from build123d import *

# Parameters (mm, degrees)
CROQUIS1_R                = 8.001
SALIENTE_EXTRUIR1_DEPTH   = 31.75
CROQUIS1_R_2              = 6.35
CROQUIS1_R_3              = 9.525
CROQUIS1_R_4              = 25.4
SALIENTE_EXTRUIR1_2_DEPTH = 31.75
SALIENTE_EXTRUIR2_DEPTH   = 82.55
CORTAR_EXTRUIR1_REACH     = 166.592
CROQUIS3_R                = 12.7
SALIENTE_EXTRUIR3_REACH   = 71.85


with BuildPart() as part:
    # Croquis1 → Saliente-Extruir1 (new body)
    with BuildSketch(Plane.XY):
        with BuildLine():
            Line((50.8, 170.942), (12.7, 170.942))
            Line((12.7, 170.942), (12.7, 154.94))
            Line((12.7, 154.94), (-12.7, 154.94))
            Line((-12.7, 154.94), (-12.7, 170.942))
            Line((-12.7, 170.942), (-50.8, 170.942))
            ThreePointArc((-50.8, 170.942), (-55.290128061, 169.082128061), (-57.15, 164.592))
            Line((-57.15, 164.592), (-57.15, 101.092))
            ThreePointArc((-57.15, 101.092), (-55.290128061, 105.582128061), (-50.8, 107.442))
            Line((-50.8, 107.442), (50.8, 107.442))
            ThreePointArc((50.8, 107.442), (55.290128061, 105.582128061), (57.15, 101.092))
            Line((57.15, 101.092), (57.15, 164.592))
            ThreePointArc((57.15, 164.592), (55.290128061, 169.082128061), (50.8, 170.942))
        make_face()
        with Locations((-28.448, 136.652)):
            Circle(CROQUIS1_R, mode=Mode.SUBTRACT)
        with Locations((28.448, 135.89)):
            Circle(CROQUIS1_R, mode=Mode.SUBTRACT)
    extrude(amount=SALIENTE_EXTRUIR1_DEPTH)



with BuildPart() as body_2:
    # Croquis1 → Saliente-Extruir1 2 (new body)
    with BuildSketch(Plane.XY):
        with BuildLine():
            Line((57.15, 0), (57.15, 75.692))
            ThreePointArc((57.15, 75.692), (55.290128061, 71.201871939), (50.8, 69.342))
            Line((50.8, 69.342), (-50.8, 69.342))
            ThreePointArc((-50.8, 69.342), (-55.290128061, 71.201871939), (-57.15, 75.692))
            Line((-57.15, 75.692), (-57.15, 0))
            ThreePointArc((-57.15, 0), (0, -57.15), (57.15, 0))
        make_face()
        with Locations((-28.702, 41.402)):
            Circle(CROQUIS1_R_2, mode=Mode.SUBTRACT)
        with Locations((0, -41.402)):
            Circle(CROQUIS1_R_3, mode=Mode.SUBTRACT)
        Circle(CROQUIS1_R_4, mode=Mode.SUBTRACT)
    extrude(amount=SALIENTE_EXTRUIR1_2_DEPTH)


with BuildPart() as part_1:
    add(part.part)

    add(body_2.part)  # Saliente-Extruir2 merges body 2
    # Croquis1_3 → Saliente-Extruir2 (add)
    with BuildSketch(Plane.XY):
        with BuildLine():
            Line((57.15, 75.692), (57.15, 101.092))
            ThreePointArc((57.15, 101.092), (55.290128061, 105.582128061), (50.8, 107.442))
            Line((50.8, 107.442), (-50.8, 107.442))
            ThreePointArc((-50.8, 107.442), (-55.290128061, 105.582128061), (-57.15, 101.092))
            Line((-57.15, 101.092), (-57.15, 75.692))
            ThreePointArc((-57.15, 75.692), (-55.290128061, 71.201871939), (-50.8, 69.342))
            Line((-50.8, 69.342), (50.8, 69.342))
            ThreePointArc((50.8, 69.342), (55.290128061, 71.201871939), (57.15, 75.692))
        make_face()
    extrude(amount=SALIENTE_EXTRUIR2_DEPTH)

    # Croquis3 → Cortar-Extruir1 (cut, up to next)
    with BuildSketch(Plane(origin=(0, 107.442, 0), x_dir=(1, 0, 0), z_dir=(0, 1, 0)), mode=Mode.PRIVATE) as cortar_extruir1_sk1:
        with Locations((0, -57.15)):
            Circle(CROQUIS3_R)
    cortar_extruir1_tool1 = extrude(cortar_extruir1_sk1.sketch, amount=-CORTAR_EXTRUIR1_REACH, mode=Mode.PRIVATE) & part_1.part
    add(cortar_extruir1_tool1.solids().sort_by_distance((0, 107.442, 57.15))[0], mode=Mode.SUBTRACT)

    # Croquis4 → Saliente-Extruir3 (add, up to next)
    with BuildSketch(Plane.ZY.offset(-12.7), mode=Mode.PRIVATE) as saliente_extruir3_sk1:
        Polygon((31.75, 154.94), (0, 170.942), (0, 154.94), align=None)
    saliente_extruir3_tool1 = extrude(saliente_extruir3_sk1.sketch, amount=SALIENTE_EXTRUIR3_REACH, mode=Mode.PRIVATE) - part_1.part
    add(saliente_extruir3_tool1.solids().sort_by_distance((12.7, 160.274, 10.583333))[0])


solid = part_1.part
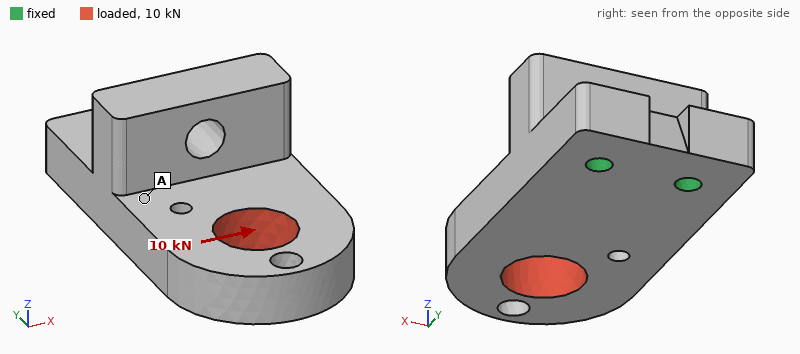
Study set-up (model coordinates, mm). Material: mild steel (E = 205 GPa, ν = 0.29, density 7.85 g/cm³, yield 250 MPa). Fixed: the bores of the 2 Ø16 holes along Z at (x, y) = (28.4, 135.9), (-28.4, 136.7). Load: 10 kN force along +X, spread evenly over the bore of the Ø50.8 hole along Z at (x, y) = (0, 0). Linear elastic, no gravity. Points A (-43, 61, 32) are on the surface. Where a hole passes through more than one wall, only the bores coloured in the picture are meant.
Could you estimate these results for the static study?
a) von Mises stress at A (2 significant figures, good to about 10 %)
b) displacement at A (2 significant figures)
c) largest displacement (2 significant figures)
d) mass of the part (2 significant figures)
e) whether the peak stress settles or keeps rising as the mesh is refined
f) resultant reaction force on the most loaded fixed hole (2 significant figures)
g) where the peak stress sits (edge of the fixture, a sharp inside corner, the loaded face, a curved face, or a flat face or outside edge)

7.1 MPa
9.3 µm
31 µm
7.0 kg
keeps rising
21 kN
edge of the fixture
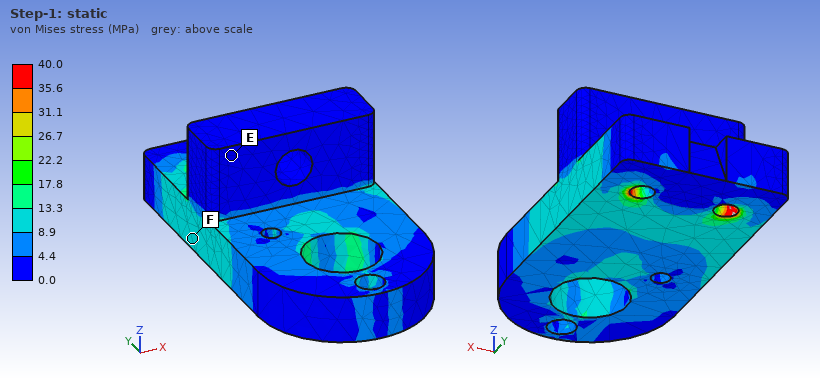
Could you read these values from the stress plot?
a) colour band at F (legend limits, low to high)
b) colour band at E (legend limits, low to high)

8.9 to 13.3 MPa
0.0 to 4.4 MPa
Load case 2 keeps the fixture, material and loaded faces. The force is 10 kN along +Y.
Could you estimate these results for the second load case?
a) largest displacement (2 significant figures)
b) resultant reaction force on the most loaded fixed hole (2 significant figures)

4.0 µm
5.0 kN
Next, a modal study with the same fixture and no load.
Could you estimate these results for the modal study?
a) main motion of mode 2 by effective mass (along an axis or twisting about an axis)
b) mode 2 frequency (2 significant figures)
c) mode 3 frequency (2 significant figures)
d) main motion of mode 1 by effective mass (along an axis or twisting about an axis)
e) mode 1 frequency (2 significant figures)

along X
2200 Hz
2600 Hz
along Z
880 Hz
